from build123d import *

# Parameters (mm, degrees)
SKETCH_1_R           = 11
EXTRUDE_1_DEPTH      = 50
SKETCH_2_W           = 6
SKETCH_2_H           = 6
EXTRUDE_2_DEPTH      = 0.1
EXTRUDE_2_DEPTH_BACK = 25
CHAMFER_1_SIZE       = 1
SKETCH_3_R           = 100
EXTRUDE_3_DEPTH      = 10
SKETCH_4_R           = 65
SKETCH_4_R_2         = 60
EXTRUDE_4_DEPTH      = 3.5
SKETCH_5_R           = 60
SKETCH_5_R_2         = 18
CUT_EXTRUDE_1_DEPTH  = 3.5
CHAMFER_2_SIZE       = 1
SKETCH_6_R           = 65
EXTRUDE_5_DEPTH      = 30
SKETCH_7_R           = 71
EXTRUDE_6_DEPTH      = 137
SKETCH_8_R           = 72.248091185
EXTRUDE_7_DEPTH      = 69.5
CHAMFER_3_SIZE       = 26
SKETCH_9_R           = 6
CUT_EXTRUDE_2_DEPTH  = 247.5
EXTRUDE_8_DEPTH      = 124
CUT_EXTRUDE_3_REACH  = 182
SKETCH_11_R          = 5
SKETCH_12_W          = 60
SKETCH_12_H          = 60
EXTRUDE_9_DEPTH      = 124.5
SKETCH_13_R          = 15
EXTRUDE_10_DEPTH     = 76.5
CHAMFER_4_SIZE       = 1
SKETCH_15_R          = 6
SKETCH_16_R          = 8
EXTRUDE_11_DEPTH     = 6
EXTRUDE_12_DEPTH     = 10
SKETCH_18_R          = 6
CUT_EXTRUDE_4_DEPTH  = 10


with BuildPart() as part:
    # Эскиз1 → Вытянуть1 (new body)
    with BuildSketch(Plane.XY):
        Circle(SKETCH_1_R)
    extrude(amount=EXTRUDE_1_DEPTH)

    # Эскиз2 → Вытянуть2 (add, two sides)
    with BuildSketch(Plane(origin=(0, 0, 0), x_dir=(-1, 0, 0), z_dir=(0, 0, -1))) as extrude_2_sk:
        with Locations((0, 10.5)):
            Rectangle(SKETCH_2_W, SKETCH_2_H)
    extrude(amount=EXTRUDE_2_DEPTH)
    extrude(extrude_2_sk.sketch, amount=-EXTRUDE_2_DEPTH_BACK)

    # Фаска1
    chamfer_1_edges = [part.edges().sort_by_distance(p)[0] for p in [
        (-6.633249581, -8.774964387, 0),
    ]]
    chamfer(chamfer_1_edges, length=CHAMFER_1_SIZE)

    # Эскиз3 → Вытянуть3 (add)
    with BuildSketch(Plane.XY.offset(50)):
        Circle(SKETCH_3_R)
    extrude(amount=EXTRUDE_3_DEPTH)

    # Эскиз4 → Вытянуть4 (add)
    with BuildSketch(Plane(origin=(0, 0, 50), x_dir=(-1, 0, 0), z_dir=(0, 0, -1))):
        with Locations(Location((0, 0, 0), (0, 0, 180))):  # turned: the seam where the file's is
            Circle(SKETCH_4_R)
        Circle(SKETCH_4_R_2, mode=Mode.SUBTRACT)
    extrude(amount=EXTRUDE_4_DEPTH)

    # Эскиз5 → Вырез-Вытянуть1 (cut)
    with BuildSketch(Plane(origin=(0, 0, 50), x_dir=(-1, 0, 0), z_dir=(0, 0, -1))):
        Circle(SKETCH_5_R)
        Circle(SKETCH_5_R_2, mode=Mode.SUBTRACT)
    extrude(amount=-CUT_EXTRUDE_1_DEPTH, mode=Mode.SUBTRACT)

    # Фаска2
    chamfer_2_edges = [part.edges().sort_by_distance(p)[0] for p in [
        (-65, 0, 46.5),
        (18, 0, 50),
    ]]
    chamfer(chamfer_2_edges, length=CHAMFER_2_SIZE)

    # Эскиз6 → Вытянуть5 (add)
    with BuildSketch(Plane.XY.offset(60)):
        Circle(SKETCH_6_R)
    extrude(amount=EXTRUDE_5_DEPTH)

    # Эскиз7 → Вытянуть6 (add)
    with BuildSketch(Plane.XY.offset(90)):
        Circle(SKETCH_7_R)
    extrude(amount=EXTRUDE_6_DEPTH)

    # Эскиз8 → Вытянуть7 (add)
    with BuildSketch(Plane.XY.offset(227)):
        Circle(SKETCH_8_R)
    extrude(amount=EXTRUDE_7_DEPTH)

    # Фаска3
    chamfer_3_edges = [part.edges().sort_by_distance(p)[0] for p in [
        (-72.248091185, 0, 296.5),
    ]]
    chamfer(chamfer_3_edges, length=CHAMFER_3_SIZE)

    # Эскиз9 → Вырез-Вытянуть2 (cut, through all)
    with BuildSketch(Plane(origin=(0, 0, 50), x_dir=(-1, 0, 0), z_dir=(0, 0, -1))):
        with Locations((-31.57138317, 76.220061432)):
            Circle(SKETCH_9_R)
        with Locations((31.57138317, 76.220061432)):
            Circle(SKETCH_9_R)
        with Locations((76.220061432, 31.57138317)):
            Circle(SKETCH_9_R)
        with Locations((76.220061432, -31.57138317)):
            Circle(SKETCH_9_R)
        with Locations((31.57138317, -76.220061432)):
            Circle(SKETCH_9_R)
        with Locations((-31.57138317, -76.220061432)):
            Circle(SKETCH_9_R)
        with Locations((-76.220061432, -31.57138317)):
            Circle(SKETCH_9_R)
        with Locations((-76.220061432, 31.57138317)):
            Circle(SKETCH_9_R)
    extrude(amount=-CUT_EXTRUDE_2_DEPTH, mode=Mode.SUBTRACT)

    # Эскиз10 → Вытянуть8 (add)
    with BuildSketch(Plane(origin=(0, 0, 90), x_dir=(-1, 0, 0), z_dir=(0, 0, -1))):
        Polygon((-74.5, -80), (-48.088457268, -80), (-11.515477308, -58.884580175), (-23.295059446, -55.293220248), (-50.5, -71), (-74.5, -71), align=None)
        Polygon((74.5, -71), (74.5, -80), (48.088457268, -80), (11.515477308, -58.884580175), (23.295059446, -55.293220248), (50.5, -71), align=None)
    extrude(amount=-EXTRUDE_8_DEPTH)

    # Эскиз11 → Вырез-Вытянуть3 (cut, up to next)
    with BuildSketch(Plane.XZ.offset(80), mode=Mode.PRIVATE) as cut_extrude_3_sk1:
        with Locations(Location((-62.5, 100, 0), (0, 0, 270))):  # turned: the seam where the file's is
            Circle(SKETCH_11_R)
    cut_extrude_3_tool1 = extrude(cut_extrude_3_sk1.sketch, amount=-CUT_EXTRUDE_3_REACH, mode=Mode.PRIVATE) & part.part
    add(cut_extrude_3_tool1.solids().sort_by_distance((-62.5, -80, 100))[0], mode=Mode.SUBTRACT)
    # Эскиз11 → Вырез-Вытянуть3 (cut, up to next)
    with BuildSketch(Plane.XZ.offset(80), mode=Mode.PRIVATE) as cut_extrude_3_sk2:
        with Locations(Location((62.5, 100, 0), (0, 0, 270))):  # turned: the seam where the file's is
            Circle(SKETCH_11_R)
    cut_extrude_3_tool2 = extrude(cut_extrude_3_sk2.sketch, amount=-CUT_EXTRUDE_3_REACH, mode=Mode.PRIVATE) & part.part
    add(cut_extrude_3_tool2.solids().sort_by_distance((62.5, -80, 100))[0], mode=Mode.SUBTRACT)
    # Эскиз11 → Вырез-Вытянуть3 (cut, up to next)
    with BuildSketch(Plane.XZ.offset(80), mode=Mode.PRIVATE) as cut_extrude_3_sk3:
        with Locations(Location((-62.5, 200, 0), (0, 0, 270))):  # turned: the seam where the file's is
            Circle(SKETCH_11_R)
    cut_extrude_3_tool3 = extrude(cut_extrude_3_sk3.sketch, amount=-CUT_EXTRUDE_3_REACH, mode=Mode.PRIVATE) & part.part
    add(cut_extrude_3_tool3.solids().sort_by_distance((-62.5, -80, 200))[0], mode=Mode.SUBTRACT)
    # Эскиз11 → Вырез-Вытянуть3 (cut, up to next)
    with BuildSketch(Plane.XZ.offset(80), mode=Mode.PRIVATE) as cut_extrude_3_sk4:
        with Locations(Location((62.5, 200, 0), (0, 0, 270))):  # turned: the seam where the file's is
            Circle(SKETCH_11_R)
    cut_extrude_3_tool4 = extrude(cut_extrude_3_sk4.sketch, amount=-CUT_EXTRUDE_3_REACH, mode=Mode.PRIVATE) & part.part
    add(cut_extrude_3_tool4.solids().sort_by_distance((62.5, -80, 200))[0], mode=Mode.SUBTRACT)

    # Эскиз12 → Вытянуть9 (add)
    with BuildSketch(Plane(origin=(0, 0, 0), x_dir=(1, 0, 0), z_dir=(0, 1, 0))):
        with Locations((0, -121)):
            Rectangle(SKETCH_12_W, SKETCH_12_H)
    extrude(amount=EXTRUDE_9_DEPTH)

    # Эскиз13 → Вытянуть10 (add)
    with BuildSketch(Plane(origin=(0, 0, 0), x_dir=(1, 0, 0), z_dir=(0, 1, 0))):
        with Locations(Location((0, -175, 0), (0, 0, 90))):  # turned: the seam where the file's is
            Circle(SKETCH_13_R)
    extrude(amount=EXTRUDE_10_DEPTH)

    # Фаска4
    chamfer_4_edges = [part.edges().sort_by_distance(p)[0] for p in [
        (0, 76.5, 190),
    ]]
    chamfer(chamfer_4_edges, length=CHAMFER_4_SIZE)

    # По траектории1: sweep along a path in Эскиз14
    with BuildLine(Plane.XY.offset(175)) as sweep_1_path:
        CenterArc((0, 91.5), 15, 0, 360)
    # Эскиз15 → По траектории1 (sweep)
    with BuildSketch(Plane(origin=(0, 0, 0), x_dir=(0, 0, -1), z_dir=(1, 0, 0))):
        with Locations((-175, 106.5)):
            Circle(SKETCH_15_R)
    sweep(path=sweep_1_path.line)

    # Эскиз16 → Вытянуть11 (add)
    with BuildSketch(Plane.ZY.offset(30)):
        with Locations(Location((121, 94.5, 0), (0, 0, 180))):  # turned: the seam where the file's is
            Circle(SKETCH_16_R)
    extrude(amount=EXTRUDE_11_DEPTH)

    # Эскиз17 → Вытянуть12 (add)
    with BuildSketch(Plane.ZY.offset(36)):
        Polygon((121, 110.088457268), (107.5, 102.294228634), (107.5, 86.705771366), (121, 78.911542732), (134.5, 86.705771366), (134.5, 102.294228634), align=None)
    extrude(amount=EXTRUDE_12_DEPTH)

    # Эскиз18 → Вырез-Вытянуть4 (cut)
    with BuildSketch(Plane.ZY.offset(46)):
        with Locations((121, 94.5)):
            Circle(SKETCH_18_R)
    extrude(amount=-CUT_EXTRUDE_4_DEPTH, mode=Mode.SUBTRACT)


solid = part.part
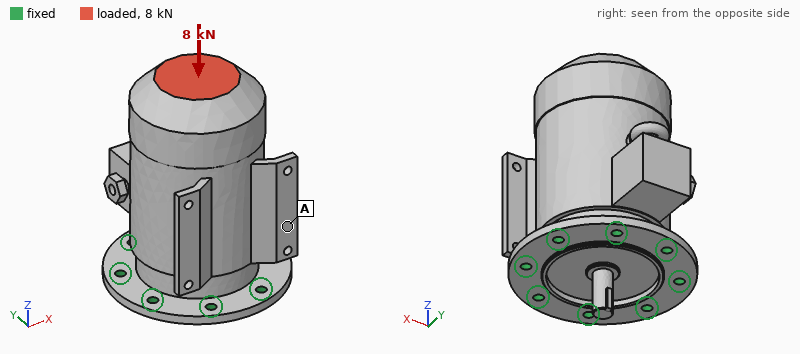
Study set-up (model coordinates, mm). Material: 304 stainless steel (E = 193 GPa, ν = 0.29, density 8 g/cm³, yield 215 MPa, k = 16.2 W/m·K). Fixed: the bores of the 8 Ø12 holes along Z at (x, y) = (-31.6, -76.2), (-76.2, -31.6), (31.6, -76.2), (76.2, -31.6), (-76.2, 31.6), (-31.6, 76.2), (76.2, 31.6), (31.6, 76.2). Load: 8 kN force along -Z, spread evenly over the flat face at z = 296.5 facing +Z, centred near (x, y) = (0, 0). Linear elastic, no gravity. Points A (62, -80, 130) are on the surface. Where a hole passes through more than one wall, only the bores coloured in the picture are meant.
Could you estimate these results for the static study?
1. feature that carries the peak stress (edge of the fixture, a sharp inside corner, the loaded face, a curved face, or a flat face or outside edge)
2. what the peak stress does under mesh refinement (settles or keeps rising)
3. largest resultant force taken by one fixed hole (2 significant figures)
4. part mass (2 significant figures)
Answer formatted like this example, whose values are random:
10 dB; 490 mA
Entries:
edge of the fixture; keeps rising; 1.2 kN; 34 kg
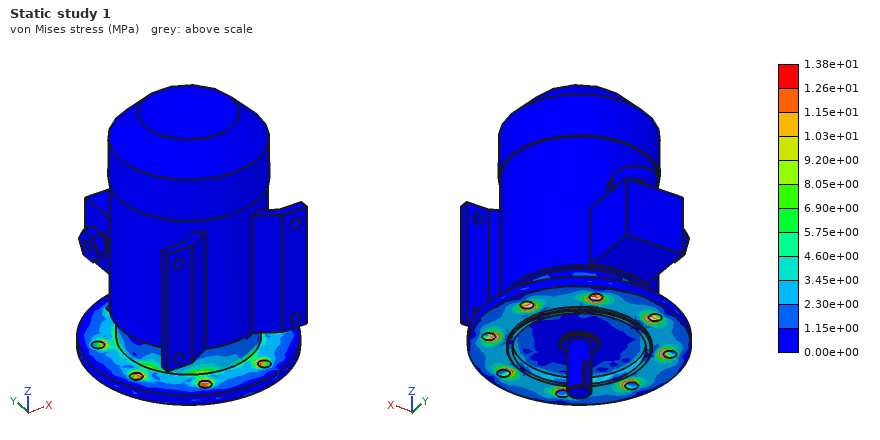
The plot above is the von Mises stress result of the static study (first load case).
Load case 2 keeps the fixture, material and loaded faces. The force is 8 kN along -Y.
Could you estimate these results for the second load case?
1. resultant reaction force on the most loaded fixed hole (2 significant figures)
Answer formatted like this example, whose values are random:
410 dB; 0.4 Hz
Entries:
6.7 kN
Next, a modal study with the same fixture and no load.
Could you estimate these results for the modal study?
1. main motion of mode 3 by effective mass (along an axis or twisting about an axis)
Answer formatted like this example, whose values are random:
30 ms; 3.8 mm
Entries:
along Z
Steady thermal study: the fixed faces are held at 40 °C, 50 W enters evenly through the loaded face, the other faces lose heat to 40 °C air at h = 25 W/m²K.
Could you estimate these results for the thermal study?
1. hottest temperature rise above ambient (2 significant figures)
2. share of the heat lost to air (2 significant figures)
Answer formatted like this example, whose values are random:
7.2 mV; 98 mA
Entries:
35 K; 85 %
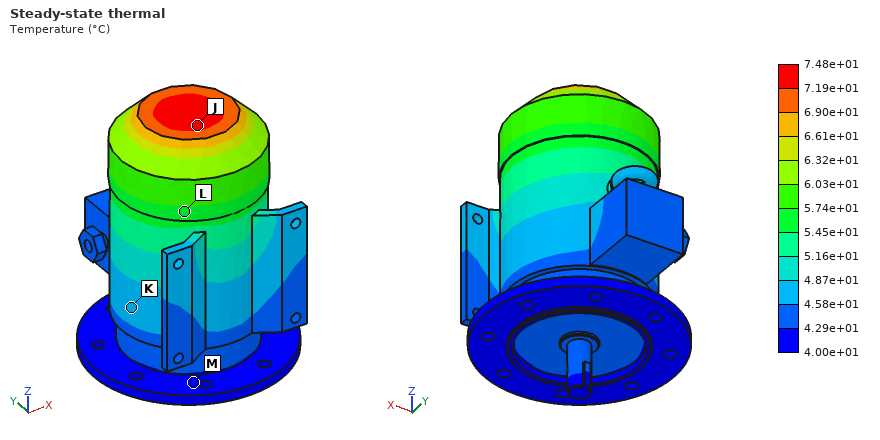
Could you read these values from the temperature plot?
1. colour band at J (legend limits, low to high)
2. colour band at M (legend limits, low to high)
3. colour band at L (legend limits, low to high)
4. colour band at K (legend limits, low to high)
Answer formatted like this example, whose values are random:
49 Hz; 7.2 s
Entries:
7.19e+01 to 7.48e+01 °C; 4.00e+01 to 4.29e+01 °C; 5.45e+01 to 5.74e+01 °C; 4.58e+01 to 4.87e+01 °C
